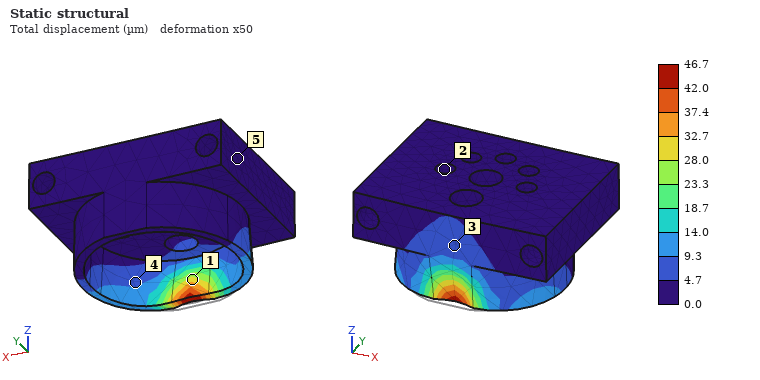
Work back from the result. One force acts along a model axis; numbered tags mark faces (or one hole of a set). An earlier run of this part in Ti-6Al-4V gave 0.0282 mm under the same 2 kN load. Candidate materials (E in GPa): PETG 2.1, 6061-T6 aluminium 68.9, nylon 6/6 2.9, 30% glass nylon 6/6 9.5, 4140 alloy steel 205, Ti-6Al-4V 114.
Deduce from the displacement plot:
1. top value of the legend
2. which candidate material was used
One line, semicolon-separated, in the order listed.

46.7 µm; 6061-T6 aluminium
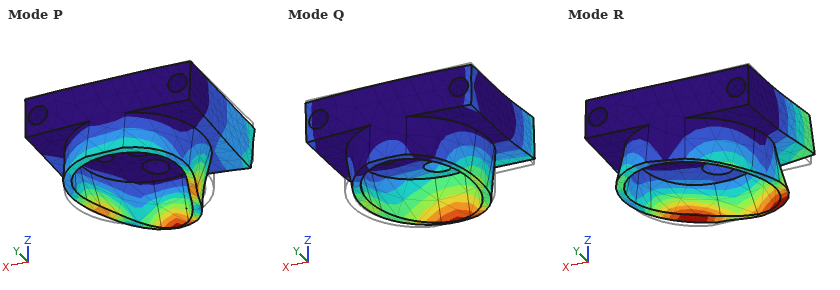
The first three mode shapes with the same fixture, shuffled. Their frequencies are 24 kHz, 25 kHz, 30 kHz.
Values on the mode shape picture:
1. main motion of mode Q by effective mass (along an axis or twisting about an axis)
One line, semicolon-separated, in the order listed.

along Z
